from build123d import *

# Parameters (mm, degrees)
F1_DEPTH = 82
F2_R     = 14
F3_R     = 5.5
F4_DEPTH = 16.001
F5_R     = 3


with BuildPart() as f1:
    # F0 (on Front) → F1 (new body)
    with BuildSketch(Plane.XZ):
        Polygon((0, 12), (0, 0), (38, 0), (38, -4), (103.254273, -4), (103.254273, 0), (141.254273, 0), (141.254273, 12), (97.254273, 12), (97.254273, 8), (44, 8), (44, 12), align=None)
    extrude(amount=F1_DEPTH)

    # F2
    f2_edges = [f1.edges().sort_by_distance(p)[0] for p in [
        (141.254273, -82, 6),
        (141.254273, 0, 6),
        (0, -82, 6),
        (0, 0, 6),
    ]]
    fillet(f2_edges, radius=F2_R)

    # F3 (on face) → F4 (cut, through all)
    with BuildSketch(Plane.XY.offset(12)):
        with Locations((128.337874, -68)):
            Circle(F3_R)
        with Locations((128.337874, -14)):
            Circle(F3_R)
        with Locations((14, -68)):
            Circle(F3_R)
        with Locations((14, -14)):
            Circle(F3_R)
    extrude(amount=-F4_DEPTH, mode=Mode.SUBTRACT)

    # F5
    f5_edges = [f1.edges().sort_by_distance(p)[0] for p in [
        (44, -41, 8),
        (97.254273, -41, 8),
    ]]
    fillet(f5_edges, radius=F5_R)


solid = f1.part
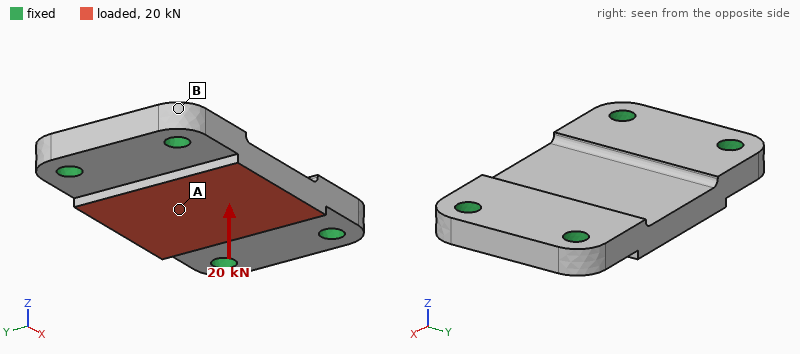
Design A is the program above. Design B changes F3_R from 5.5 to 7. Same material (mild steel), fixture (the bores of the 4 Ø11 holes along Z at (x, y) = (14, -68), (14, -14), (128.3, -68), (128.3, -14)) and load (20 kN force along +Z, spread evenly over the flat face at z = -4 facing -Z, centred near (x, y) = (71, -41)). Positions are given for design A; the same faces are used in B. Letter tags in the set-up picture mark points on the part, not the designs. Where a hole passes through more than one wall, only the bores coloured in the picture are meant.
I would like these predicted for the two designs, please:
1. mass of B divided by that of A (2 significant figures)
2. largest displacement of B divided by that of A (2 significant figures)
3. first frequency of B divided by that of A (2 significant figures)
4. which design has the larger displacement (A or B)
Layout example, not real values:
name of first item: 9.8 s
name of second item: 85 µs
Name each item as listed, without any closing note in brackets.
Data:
mass of B divided by that of A: 0.98
largest displacement of B divided by that of A: 0.88
first frequency of B divided by that of A: 1.1
which design has the larger displacement: A
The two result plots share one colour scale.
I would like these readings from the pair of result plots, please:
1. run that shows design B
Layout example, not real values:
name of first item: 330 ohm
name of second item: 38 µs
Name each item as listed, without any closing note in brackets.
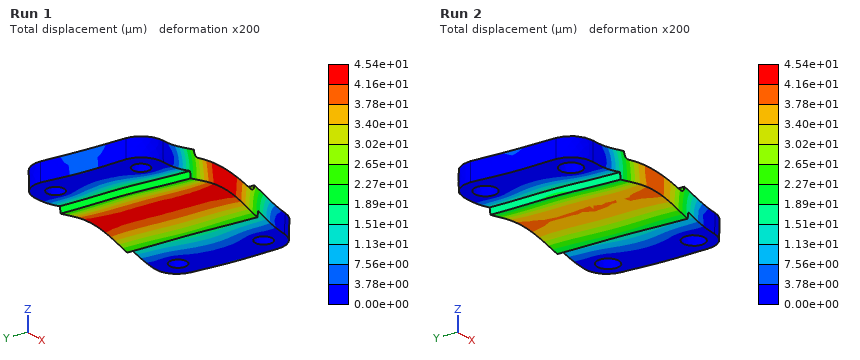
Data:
run that shows design B: Run 2
